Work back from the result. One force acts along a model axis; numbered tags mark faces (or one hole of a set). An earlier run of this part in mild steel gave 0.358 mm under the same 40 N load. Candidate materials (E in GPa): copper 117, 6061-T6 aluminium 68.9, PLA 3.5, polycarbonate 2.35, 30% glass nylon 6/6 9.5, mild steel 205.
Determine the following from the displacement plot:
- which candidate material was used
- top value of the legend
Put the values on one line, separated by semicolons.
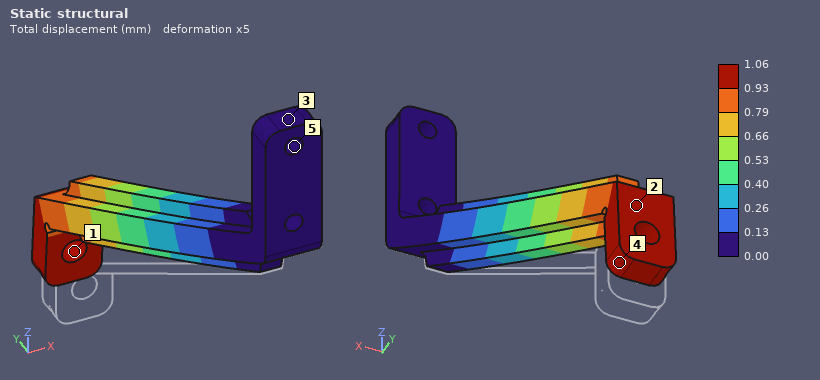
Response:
6061-T6 aluminium; 1.06 mm
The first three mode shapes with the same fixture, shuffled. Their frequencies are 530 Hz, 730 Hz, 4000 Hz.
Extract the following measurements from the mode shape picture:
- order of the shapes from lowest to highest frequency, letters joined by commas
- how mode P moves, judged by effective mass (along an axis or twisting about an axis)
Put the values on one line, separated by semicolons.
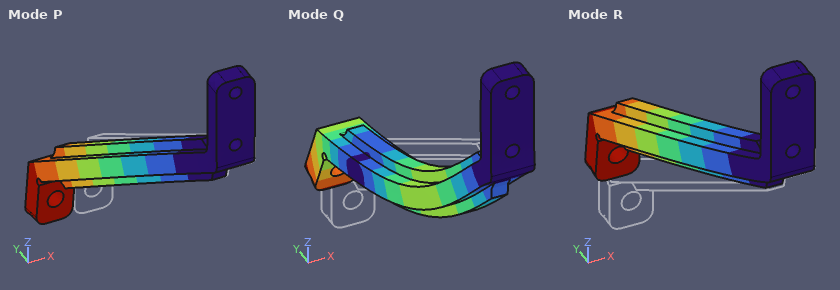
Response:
R, P, Q; along X
